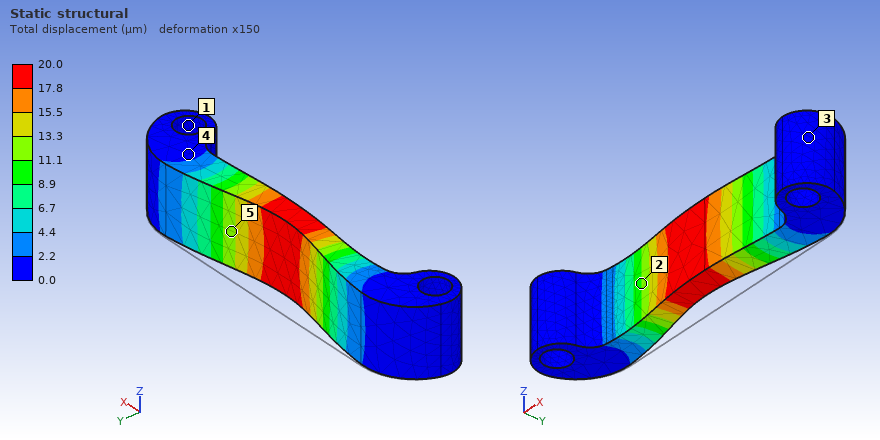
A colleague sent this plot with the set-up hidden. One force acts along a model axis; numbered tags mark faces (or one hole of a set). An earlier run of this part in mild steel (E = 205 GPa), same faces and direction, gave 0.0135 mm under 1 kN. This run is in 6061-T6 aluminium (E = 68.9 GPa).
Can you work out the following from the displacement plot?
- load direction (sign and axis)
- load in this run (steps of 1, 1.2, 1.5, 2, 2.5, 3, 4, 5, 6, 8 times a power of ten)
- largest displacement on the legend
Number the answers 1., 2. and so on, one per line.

1. -Y
2. 500 N
3. 20.0 µm
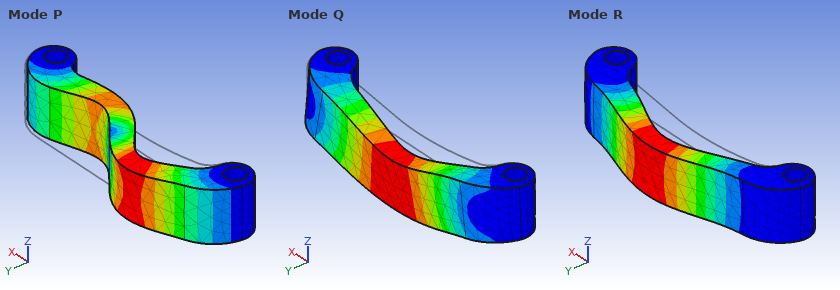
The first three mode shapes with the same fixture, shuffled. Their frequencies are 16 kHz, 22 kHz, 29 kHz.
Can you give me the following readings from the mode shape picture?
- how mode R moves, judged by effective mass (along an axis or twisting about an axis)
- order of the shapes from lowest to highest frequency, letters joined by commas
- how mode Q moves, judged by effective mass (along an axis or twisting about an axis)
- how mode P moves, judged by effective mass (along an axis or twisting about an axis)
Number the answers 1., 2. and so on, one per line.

1. along Y
2. R, Q, P
3. along Z
4. along X
